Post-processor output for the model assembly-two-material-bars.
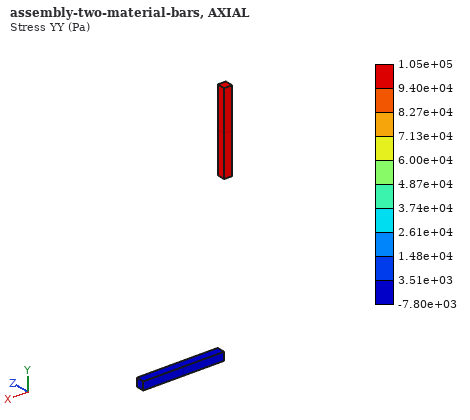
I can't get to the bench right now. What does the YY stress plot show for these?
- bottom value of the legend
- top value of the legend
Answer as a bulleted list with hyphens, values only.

- -7.80e+03 Pa
- 1.05e+05 Pa
